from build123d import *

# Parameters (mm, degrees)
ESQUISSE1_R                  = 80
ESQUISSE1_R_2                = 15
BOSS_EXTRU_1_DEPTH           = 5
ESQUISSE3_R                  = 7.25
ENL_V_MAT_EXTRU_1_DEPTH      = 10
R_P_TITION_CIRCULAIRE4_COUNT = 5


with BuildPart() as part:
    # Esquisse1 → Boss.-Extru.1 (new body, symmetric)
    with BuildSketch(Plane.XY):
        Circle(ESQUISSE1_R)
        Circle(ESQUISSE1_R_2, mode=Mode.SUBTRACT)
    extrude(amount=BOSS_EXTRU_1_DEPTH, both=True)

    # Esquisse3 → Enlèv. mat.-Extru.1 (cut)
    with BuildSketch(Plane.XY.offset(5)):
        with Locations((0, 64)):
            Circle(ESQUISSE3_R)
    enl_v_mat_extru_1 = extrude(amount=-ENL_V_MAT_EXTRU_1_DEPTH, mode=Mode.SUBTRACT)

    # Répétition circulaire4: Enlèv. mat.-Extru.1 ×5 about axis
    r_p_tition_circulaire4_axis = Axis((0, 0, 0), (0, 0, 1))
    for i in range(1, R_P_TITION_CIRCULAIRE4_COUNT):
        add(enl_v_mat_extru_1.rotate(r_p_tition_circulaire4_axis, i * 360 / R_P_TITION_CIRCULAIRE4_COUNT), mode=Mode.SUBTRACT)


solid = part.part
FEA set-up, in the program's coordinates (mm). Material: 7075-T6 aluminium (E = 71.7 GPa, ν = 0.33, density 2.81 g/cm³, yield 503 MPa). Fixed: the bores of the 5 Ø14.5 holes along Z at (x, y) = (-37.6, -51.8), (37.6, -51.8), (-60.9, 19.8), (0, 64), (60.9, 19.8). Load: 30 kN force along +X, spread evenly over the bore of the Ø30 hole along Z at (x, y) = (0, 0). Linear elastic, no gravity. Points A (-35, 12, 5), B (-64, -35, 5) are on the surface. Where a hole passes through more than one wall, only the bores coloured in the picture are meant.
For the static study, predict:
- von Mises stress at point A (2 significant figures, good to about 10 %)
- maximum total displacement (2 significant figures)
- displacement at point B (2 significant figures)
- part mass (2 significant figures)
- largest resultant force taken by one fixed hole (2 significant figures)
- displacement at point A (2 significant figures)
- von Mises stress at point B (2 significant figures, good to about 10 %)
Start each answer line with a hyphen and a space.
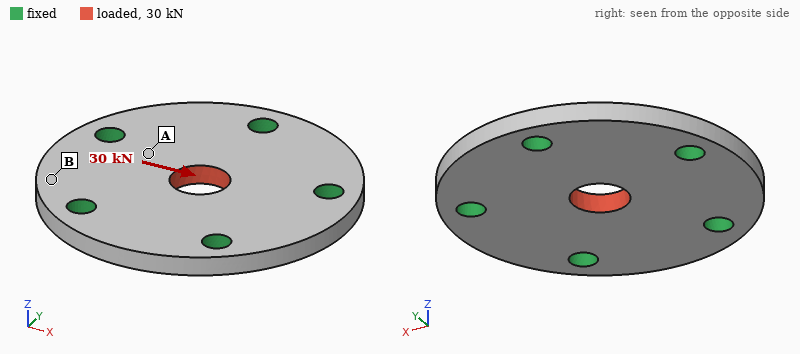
- 29 MPa
- 19 µm
- 6.1 µm
- 520 g
- 8.5 kN
- 8.5 µm
- 7.5 MPa
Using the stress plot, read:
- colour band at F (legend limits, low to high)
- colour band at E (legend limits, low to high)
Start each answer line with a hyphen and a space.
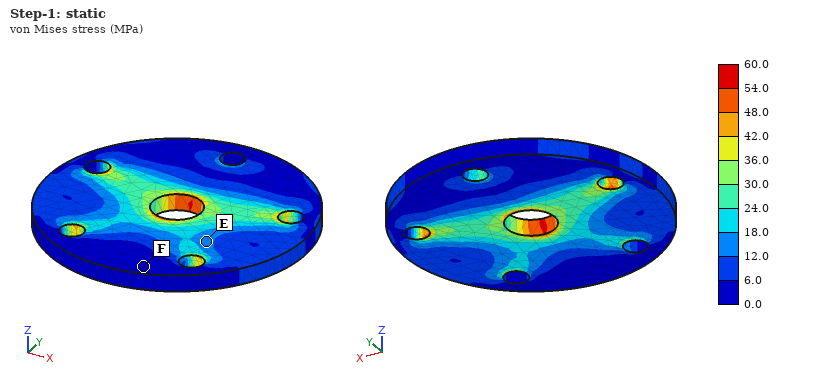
- 0.0 to 6.0 MPa
- 12.0 to 18.0 MPa
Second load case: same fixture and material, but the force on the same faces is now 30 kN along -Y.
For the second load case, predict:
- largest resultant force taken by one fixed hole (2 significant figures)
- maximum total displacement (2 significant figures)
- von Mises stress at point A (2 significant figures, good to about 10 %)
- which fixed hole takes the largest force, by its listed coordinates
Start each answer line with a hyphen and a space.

- 8.8 kN
- 19 µm
- 11 MPa
- (0, 64)
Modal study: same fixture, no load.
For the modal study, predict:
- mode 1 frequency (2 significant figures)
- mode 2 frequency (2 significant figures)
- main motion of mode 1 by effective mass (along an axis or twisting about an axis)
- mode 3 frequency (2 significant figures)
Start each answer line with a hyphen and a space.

- 5700 Hz
- 8100 Hz
- along Z
- 8100 Hz
